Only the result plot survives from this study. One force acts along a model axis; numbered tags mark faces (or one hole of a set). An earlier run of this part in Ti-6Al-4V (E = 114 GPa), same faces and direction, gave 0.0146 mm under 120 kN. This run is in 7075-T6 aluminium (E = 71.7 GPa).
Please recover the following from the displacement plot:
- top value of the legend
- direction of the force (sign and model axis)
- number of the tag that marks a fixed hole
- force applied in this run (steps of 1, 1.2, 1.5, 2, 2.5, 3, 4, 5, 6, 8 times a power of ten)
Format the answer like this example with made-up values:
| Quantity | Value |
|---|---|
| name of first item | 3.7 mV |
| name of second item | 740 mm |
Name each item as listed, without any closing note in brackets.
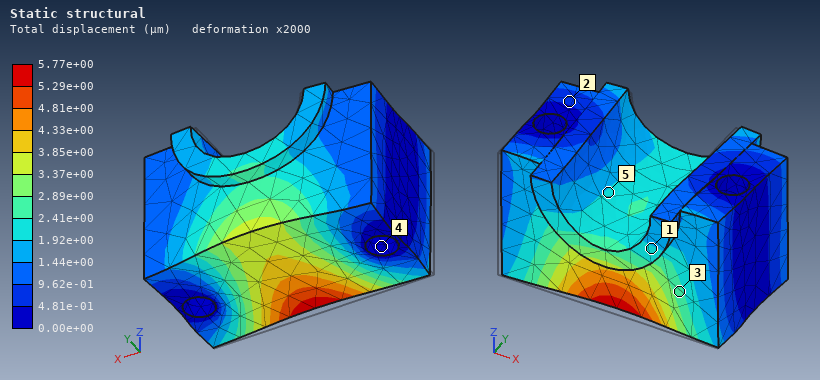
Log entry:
| Quantity | Value |
|---|---|
| top value of the legend | 5.77e+00 µm |
| direction of the force | +Y |
| number of the tag that marks a fixed hole | 4 |
| force applied in this run | 30 kN |
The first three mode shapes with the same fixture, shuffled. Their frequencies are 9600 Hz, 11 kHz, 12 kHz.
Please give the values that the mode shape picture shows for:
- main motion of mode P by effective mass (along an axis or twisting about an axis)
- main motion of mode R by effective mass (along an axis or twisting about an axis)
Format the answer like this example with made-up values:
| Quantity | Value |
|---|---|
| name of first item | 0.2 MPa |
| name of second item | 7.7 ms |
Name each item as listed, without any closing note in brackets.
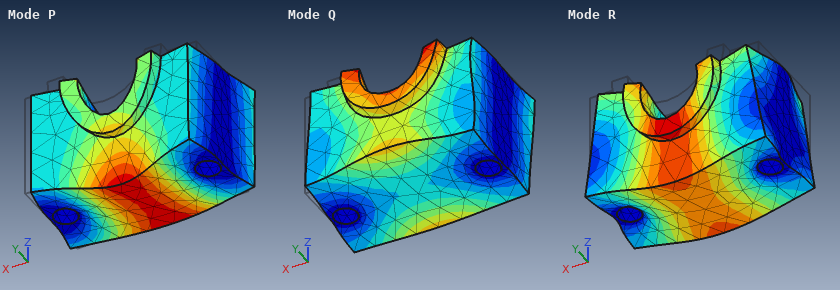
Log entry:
| Quantity | Value |
|---|---|
| main motion of mode P by effective mass | along Y |
| main motion of mode R by effective mass | along Z |
